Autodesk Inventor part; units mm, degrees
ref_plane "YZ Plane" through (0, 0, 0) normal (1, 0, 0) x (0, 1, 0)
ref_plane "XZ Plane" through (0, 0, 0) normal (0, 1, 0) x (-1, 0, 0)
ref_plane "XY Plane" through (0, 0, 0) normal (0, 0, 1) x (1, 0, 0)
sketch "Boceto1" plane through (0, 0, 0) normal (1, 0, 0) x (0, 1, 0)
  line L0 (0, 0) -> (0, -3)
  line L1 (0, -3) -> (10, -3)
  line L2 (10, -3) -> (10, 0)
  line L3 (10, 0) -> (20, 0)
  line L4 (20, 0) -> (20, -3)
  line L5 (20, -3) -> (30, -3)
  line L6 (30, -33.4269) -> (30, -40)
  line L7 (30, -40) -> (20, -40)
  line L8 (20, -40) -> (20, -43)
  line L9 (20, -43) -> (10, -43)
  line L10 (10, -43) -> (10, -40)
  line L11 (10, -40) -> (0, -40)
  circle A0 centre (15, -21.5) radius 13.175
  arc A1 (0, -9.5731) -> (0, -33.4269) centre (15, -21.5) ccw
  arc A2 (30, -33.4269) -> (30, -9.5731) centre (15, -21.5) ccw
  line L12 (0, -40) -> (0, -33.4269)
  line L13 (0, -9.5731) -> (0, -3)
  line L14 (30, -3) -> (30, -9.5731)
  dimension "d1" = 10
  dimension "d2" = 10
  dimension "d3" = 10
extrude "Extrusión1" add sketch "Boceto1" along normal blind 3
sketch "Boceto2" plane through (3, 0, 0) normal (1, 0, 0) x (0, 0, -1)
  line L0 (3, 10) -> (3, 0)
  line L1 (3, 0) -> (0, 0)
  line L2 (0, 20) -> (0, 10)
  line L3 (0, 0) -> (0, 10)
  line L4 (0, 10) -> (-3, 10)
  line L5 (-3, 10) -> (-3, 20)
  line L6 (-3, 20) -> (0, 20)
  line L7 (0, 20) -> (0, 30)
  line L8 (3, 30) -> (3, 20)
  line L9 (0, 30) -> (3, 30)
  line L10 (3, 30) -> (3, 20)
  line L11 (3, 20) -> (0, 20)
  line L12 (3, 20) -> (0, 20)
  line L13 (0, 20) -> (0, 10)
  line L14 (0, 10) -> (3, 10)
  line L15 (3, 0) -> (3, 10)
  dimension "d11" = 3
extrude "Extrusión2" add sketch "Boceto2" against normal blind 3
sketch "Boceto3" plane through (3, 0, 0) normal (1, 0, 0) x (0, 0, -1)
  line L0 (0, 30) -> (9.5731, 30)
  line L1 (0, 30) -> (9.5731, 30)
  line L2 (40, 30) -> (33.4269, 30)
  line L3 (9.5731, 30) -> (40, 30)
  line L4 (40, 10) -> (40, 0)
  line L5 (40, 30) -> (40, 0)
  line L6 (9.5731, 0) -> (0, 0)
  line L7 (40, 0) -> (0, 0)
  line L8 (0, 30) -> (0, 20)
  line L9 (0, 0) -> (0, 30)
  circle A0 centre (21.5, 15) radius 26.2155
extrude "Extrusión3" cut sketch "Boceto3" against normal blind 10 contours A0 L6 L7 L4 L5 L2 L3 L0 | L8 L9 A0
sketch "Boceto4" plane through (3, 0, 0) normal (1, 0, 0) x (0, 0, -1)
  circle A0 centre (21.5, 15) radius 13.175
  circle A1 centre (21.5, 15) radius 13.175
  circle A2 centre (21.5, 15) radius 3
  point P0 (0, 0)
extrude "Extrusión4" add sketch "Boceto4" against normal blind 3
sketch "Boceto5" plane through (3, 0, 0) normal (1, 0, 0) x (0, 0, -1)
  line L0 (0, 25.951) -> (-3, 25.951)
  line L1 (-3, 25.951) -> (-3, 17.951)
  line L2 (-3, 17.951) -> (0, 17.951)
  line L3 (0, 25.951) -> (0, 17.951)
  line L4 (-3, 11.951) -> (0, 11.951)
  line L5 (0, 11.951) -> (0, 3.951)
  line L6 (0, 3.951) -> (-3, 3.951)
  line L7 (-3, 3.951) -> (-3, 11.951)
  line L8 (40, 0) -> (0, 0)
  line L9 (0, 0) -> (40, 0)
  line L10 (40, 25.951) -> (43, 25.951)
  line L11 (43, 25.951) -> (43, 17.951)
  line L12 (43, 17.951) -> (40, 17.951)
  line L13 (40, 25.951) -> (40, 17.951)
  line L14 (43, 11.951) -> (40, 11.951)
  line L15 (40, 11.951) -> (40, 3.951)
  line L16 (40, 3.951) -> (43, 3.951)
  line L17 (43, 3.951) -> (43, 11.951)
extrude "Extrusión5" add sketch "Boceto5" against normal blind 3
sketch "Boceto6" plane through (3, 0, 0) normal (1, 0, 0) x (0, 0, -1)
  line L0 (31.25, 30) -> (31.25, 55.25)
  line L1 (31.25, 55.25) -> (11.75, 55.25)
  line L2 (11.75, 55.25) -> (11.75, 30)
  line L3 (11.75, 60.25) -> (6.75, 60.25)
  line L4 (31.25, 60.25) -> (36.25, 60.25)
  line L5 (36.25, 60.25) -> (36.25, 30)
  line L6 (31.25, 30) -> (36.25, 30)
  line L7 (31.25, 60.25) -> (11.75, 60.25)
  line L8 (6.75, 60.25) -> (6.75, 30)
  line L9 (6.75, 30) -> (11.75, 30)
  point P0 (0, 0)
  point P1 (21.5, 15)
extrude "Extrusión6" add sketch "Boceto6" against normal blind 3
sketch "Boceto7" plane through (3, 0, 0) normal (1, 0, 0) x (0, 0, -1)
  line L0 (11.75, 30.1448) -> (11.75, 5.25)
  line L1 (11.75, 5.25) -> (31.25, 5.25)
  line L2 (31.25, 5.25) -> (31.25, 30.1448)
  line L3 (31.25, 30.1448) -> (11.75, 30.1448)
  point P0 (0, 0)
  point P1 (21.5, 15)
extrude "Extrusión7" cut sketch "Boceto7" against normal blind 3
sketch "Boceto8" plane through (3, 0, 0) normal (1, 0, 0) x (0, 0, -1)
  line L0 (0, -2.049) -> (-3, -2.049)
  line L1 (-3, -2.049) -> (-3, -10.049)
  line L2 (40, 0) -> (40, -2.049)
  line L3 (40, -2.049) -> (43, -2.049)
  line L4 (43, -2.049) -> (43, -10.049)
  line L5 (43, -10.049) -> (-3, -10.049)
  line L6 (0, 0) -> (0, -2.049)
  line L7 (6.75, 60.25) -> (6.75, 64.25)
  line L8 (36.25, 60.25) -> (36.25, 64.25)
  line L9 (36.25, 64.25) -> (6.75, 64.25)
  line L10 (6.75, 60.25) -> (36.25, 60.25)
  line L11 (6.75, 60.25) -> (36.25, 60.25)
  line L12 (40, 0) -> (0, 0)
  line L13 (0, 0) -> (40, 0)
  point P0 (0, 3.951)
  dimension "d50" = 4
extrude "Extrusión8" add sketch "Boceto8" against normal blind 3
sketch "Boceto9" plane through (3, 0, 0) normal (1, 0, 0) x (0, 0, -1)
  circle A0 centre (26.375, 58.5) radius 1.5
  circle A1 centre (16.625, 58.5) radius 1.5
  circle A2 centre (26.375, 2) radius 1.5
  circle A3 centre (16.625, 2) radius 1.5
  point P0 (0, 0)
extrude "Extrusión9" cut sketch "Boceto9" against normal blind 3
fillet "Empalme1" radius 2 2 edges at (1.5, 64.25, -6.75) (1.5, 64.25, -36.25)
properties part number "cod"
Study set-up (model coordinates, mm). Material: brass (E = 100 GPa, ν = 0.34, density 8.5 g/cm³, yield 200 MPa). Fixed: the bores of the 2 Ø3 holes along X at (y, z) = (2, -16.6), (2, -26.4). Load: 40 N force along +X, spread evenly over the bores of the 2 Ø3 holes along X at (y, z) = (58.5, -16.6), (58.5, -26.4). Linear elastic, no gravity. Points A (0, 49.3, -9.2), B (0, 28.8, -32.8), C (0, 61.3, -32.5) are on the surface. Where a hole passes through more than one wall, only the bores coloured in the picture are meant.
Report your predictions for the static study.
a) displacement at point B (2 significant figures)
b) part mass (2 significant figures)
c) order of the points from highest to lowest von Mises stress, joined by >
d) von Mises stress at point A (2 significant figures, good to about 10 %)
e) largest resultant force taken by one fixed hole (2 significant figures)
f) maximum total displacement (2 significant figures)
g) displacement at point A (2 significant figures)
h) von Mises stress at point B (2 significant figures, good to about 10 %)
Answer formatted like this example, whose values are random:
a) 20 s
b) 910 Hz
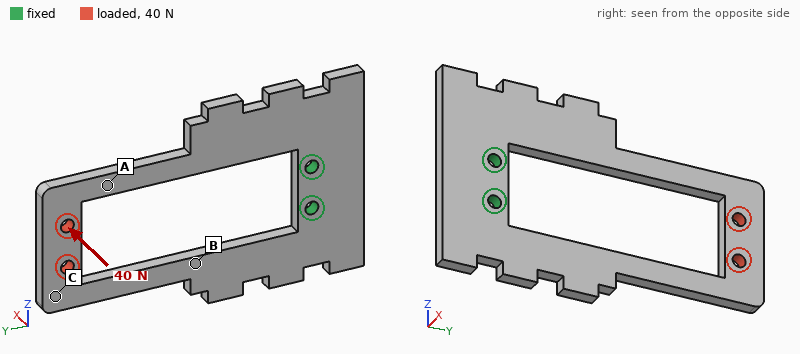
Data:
a) 0.21 mm
b) 45 g
c) B > A > C
d) 26 MPa
e) 21 N
f) 0.85 mm
g) 0.53 mm
h) 62 MPa
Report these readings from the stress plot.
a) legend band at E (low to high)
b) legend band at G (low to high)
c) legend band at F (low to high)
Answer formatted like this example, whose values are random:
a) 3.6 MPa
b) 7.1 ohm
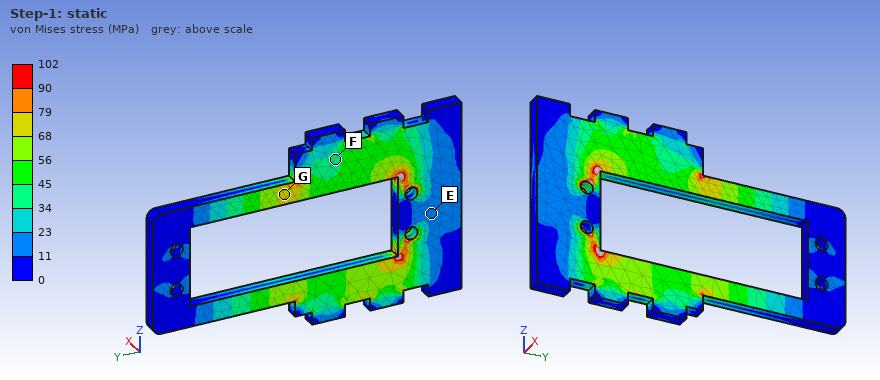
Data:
a) 11 to 23 MPa
b) 68 to 79 MPa
c) 34 to 45 MPa
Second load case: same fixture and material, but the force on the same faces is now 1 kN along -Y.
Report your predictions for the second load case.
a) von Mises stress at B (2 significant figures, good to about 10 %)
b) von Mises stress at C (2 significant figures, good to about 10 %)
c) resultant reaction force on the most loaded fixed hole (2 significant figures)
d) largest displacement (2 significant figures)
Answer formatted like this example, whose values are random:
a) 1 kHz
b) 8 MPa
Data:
a) 29 MPa
b) 20 MPa
c) 630 N
d) 37 µm
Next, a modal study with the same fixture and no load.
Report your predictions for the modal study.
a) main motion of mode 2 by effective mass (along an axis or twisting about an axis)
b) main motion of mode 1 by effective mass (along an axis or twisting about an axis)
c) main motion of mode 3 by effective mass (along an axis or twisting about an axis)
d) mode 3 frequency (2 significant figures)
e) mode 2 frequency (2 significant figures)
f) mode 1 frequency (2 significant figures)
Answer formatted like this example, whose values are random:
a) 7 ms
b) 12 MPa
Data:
a) twisting about Y
b) along X
c) along Z
d) 1500 Hz
e) 1100 Hz
f) 380 Hz
